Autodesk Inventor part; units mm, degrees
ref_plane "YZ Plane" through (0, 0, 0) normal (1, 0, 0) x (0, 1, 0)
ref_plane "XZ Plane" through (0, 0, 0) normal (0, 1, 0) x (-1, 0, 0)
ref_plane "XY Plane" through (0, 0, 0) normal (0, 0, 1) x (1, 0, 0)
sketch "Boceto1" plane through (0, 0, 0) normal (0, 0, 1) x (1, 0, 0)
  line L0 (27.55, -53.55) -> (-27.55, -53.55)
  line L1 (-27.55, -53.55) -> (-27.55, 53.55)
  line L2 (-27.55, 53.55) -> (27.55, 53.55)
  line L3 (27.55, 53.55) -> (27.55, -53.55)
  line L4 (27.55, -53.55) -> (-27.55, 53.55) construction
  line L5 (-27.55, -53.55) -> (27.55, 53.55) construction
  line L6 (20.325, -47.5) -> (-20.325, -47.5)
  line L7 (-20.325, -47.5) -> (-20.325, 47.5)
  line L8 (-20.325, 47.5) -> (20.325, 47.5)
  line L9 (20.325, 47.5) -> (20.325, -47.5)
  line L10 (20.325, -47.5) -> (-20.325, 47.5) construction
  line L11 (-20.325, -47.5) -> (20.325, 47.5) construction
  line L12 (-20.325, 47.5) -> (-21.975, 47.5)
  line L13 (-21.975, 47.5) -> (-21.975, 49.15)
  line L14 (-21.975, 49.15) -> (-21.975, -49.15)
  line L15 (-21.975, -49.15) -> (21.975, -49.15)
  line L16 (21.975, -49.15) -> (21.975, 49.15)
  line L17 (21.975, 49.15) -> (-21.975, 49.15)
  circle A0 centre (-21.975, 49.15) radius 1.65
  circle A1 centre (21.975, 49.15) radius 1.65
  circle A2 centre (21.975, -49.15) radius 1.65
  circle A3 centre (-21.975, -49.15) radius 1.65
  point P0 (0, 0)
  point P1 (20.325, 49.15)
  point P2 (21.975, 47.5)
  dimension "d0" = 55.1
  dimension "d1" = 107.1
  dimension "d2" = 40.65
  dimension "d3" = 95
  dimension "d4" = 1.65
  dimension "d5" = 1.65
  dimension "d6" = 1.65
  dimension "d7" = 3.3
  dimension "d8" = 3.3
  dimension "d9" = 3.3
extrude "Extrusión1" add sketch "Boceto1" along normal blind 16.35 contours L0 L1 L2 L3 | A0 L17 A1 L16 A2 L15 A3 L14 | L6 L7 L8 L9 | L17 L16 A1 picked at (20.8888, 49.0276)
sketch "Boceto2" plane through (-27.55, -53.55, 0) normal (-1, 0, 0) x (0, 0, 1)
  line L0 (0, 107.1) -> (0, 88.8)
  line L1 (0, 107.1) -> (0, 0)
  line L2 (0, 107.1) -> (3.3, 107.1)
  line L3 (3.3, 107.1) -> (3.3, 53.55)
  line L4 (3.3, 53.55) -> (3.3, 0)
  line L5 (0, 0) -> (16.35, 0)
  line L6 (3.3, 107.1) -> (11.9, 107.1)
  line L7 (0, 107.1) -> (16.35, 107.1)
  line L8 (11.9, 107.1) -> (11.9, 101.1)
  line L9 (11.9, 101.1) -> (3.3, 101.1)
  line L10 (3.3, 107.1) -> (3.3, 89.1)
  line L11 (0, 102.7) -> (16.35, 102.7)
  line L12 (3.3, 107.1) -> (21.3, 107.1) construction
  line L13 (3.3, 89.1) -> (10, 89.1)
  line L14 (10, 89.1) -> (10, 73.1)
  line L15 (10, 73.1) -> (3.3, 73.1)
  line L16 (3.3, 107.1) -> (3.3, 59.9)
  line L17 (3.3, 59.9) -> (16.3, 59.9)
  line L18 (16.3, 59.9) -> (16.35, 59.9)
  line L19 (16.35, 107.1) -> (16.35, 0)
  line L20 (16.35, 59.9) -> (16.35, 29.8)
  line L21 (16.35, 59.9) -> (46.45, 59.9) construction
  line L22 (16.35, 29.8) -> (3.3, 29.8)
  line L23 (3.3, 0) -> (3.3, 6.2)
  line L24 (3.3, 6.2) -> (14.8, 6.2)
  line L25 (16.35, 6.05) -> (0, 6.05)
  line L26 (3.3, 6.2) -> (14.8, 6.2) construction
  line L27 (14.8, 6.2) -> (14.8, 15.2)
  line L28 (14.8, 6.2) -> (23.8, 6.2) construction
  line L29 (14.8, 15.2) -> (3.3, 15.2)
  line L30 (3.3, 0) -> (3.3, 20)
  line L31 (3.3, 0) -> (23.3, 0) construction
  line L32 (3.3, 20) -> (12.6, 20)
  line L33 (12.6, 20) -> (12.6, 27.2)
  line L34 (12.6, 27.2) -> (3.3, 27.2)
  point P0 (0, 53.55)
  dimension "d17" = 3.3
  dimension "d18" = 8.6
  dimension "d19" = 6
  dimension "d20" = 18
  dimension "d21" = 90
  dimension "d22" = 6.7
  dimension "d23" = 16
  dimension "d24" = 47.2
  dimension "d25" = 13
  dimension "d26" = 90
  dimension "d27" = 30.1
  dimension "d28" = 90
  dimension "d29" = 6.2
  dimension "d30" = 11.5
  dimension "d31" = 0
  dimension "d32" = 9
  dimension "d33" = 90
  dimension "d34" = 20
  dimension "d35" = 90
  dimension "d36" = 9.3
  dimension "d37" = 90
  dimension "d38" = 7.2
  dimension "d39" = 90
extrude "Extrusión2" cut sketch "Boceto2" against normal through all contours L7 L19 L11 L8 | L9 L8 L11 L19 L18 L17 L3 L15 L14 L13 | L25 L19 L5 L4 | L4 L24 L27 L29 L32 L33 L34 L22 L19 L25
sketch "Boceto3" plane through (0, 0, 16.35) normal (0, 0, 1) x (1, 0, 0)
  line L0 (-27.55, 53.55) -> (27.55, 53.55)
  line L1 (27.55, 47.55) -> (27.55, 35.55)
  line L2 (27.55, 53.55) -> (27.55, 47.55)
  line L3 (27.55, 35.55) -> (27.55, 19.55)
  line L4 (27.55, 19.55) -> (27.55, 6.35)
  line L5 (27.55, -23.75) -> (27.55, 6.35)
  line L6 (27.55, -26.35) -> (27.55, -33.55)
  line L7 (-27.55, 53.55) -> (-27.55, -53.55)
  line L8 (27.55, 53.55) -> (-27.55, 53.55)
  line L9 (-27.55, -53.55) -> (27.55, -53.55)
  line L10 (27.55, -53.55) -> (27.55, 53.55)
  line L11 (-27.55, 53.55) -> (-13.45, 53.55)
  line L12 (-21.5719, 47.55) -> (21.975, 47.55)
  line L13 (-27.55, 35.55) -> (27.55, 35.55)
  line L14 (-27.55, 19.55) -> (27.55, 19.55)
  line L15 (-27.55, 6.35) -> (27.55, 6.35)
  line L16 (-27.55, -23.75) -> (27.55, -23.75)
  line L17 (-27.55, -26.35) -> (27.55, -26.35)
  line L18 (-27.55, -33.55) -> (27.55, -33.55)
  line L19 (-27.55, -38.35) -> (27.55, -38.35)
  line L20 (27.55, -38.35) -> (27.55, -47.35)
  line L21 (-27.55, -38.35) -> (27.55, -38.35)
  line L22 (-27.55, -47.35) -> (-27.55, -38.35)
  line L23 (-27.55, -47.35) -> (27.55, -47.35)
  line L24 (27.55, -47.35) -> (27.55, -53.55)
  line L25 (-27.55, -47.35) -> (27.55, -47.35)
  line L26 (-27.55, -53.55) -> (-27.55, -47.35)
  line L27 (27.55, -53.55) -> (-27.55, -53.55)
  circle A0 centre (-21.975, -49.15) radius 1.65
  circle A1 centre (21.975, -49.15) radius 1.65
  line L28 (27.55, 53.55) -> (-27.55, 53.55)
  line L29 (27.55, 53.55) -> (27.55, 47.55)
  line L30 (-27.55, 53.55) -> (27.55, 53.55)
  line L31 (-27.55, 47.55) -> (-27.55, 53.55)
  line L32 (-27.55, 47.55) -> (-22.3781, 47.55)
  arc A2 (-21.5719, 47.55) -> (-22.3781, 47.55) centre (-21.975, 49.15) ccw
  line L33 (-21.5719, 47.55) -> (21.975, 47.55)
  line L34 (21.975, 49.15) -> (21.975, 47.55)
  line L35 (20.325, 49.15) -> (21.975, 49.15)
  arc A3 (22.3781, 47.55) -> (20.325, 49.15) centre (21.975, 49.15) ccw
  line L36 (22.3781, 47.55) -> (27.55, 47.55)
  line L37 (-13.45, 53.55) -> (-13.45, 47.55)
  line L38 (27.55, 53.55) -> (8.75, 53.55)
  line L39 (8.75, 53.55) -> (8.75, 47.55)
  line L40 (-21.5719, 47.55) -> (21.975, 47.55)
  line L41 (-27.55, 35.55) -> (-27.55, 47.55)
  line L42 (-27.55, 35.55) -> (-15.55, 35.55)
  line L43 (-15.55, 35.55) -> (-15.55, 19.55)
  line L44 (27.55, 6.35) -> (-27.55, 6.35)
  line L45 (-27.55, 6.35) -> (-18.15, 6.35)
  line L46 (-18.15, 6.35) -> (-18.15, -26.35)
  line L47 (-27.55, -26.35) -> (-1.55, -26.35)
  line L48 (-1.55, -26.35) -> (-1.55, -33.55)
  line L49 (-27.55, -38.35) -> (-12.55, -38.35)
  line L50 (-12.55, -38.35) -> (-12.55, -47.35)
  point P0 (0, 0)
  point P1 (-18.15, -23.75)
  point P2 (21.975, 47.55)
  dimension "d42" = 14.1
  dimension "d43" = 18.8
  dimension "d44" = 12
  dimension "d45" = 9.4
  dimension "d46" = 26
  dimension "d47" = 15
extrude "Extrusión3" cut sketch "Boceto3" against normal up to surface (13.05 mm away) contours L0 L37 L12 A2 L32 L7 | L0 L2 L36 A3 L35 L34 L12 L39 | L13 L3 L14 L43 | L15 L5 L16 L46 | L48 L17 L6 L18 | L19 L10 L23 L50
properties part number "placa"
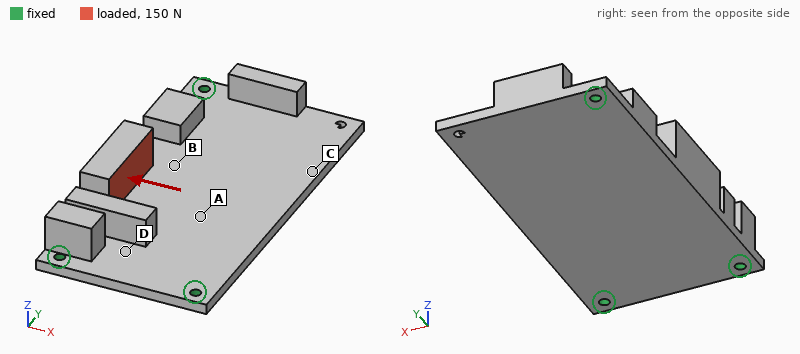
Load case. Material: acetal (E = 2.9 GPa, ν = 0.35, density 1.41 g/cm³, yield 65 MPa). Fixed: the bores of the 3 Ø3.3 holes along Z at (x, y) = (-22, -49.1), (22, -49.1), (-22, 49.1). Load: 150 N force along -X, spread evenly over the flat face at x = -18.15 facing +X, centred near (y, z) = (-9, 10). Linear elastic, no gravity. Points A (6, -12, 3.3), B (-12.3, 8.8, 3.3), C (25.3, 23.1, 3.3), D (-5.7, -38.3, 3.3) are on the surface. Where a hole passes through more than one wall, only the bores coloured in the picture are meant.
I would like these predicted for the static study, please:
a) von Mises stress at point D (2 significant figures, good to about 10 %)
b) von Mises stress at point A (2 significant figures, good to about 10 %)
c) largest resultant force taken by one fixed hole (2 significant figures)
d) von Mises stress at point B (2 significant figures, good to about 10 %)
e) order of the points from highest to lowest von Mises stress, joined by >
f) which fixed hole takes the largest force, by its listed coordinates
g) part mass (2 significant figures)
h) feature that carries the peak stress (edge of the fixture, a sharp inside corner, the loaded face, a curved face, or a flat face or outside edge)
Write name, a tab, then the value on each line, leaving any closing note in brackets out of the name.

von Mises stress at point D	4.5 MPa
von Mises stress at point A	2.4 MPa
largest resultant force taken by one fixed hole	84 N
von Mises stress at point B	3.4 MPa
order of the points from highest to lowest von Mises stress, joined by >	D > B > A > C
which fixed hole takes the largest force, by its listed coordinates	(-22, -49.1)
part mass	41 g
feature that carries the peak stress	edge of the fixture
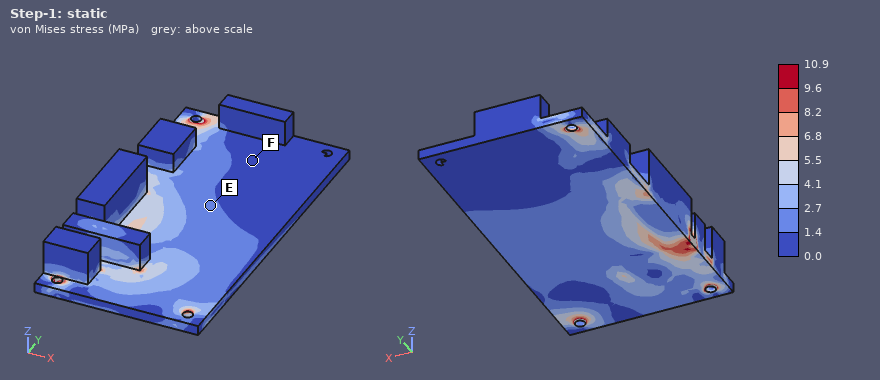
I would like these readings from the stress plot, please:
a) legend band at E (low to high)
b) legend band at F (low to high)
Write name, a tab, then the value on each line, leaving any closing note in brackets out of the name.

legend band at E	1.4 to 2.7 MPa
legend band at F	0.0 to 1.4 MPa
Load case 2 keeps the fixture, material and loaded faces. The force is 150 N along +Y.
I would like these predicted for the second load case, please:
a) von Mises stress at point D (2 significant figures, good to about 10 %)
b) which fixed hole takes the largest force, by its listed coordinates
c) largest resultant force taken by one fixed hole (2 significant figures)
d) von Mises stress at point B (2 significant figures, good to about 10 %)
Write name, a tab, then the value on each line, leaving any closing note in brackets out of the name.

von Mises stress at point D	1.4 MPa
which fixed hole takes the largest force, by its listed coordinates	(-22, -49.1)
largest resultant force taken by one fixed hole	77 N
von Mises stress at point B	5.1 MPa
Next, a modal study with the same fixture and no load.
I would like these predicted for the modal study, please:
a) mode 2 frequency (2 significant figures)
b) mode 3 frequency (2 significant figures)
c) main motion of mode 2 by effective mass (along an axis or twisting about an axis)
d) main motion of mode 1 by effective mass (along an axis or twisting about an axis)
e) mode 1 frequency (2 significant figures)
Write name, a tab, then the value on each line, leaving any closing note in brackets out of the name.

mode 2 frequency	470 Hz
mode 3 frequency	790 Hz
main motion of mode 2 by effective mass	along Z
main motion of mode 1 by effective mass	along Z
mode 1 frequency	300 Hz
